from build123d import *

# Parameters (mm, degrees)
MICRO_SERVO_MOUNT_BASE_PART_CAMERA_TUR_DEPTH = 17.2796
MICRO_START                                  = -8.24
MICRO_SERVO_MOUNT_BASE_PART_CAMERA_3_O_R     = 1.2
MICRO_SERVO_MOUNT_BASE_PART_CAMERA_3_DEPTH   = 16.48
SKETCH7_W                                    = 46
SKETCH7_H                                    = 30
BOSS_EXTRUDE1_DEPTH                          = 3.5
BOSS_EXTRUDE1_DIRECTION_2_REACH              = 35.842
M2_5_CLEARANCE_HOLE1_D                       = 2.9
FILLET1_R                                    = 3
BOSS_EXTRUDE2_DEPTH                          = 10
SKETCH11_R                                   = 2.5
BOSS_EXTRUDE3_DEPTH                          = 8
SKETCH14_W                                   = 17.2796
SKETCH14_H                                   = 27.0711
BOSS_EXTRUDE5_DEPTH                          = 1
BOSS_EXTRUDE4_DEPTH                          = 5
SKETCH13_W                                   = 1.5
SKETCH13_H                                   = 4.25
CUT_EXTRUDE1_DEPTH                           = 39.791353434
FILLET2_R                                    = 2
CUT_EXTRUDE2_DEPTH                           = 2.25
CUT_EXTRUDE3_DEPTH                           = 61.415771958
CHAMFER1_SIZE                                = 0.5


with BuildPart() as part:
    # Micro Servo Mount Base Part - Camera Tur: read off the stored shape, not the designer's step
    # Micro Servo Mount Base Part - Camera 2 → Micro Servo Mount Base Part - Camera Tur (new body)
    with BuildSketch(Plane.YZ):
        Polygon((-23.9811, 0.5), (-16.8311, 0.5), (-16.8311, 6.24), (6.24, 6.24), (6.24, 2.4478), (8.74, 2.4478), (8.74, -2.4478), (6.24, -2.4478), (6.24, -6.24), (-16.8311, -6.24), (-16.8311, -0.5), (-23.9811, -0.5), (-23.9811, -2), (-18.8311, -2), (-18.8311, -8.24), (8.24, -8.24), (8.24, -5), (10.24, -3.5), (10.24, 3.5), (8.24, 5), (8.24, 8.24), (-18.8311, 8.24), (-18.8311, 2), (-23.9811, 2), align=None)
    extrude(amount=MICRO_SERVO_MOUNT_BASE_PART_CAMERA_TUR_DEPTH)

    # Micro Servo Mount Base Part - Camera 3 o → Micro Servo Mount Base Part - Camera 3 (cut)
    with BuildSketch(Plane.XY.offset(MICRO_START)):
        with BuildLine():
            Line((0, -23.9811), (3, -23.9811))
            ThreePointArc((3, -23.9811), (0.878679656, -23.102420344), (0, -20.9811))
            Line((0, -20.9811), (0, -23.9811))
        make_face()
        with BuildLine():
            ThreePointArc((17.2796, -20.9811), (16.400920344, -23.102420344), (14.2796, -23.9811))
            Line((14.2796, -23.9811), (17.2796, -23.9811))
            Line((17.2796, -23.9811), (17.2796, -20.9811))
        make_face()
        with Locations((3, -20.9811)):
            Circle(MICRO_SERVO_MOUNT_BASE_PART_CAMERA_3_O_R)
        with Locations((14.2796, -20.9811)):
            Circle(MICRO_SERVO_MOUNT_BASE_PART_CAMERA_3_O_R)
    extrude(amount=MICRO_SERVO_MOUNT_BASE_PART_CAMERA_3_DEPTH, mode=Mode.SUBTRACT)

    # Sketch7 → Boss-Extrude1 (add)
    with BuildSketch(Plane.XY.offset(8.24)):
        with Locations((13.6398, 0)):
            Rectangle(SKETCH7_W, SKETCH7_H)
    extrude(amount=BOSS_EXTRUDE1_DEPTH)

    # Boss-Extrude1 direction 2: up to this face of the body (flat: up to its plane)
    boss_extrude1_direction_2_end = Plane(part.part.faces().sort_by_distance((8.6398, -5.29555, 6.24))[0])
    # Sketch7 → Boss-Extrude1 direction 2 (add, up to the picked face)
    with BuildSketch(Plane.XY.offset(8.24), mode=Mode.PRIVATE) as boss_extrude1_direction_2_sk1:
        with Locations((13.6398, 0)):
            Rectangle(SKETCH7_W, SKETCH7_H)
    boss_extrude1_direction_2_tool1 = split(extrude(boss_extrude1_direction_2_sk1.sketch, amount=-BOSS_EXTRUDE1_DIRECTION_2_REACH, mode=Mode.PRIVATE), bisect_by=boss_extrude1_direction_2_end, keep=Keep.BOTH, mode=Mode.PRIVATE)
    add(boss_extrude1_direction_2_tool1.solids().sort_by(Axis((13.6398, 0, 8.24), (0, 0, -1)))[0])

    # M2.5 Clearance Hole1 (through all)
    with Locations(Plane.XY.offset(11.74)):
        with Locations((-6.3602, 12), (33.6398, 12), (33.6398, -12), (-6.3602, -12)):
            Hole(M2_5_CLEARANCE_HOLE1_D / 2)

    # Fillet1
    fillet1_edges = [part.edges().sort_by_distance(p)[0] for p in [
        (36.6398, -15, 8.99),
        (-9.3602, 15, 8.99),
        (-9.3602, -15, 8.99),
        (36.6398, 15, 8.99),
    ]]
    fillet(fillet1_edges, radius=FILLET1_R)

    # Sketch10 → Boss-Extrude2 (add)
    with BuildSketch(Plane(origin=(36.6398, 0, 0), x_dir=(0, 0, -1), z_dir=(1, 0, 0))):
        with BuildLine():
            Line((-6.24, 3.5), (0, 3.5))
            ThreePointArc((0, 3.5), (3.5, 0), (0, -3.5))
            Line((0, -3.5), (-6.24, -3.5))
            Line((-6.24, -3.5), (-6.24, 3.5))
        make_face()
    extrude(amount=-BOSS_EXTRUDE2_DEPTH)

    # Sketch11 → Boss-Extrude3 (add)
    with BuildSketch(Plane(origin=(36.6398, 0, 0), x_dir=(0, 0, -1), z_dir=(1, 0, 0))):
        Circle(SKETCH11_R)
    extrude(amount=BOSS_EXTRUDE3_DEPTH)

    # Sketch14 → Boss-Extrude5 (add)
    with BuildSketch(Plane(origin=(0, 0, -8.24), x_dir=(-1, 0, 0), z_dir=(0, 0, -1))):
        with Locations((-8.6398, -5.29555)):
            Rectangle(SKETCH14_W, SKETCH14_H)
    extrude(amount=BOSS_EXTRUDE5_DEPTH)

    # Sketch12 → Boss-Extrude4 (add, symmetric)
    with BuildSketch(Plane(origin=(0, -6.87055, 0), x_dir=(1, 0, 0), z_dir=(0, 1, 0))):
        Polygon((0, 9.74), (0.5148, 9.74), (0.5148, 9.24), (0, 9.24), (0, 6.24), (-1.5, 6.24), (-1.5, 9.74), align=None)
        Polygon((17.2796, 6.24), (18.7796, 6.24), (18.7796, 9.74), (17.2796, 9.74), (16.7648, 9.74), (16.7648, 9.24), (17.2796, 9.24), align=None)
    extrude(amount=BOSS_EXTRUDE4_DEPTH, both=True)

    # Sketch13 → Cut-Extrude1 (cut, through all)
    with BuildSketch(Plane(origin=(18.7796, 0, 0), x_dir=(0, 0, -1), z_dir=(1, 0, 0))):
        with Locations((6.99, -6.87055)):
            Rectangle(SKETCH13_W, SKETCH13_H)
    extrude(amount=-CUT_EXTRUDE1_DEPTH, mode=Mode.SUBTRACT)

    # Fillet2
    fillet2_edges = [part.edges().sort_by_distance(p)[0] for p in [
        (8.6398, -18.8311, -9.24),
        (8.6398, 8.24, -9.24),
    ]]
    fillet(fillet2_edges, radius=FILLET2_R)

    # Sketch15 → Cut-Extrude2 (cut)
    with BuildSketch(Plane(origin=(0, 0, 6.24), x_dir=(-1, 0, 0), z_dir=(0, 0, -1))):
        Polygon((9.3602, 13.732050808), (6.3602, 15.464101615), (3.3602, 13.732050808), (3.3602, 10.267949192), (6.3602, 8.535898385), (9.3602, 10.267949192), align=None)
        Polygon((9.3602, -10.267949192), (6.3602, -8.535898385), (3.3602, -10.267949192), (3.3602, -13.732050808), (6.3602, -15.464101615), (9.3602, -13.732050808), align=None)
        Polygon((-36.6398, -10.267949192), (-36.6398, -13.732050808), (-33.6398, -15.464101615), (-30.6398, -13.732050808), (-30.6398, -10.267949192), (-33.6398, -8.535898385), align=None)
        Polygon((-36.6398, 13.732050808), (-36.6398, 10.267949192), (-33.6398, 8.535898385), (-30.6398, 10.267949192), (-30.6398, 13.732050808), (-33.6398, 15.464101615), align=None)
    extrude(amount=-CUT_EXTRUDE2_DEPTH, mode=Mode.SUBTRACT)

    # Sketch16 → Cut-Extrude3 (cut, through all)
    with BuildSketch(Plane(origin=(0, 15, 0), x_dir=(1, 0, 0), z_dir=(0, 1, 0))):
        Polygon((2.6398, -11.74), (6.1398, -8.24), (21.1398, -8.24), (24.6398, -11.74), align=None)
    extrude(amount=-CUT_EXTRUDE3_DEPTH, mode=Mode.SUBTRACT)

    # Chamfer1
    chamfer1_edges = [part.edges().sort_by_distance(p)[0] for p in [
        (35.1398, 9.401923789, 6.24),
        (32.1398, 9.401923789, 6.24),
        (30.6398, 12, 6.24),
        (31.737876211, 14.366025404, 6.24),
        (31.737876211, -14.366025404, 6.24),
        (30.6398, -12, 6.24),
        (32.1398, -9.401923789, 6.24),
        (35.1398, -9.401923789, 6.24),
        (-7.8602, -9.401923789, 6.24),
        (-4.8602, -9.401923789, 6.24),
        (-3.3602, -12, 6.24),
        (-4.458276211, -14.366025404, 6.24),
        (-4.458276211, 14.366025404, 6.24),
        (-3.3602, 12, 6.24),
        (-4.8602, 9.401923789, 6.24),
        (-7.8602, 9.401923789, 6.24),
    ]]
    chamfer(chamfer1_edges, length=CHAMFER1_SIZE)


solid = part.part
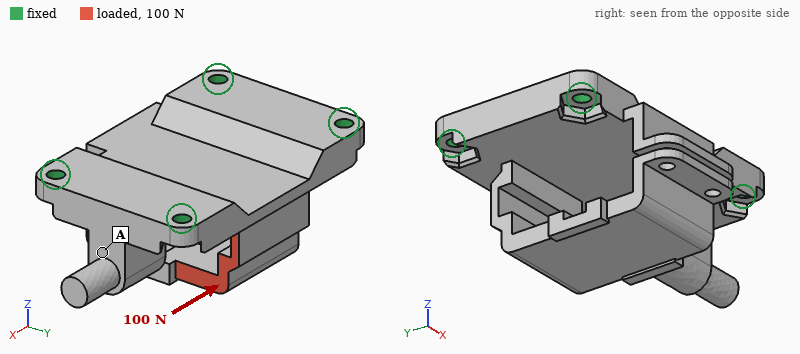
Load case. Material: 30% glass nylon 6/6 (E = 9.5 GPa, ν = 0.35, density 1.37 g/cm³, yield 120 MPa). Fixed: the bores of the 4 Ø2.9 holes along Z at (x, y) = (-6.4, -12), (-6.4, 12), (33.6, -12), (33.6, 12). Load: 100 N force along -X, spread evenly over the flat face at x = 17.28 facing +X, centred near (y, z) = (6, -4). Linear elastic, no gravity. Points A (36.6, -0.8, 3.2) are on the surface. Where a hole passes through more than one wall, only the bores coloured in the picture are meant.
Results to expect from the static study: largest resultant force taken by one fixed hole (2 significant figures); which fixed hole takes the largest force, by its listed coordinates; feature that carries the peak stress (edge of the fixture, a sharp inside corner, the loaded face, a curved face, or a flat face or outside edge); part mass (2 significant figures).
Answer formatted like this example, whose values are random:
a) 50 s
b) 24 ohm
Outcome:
a) 87 N
b) (33.6, 12)
c) the loaded face
d) 12 g
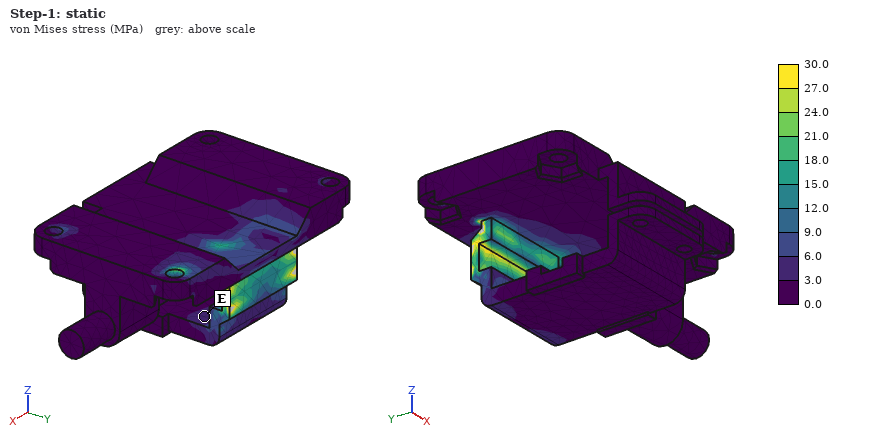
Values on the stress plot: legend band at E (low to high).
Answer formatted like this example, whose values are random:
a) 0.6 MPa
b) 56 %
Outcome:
a) 3.0 to 6.0 MPa
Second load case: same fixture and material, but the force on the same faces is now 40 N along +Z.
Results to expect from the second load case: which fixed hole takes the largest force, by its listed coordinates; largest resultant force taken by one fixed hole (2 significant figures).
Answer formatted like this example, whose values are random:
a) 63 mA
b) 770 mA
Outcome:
a) (33.6, 12)
b) 47 N
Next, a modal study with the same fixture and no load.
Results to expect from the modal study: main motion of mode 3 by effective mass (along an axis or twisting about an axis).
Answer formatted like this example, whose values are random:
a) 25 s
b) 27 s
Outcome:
a) along Y
